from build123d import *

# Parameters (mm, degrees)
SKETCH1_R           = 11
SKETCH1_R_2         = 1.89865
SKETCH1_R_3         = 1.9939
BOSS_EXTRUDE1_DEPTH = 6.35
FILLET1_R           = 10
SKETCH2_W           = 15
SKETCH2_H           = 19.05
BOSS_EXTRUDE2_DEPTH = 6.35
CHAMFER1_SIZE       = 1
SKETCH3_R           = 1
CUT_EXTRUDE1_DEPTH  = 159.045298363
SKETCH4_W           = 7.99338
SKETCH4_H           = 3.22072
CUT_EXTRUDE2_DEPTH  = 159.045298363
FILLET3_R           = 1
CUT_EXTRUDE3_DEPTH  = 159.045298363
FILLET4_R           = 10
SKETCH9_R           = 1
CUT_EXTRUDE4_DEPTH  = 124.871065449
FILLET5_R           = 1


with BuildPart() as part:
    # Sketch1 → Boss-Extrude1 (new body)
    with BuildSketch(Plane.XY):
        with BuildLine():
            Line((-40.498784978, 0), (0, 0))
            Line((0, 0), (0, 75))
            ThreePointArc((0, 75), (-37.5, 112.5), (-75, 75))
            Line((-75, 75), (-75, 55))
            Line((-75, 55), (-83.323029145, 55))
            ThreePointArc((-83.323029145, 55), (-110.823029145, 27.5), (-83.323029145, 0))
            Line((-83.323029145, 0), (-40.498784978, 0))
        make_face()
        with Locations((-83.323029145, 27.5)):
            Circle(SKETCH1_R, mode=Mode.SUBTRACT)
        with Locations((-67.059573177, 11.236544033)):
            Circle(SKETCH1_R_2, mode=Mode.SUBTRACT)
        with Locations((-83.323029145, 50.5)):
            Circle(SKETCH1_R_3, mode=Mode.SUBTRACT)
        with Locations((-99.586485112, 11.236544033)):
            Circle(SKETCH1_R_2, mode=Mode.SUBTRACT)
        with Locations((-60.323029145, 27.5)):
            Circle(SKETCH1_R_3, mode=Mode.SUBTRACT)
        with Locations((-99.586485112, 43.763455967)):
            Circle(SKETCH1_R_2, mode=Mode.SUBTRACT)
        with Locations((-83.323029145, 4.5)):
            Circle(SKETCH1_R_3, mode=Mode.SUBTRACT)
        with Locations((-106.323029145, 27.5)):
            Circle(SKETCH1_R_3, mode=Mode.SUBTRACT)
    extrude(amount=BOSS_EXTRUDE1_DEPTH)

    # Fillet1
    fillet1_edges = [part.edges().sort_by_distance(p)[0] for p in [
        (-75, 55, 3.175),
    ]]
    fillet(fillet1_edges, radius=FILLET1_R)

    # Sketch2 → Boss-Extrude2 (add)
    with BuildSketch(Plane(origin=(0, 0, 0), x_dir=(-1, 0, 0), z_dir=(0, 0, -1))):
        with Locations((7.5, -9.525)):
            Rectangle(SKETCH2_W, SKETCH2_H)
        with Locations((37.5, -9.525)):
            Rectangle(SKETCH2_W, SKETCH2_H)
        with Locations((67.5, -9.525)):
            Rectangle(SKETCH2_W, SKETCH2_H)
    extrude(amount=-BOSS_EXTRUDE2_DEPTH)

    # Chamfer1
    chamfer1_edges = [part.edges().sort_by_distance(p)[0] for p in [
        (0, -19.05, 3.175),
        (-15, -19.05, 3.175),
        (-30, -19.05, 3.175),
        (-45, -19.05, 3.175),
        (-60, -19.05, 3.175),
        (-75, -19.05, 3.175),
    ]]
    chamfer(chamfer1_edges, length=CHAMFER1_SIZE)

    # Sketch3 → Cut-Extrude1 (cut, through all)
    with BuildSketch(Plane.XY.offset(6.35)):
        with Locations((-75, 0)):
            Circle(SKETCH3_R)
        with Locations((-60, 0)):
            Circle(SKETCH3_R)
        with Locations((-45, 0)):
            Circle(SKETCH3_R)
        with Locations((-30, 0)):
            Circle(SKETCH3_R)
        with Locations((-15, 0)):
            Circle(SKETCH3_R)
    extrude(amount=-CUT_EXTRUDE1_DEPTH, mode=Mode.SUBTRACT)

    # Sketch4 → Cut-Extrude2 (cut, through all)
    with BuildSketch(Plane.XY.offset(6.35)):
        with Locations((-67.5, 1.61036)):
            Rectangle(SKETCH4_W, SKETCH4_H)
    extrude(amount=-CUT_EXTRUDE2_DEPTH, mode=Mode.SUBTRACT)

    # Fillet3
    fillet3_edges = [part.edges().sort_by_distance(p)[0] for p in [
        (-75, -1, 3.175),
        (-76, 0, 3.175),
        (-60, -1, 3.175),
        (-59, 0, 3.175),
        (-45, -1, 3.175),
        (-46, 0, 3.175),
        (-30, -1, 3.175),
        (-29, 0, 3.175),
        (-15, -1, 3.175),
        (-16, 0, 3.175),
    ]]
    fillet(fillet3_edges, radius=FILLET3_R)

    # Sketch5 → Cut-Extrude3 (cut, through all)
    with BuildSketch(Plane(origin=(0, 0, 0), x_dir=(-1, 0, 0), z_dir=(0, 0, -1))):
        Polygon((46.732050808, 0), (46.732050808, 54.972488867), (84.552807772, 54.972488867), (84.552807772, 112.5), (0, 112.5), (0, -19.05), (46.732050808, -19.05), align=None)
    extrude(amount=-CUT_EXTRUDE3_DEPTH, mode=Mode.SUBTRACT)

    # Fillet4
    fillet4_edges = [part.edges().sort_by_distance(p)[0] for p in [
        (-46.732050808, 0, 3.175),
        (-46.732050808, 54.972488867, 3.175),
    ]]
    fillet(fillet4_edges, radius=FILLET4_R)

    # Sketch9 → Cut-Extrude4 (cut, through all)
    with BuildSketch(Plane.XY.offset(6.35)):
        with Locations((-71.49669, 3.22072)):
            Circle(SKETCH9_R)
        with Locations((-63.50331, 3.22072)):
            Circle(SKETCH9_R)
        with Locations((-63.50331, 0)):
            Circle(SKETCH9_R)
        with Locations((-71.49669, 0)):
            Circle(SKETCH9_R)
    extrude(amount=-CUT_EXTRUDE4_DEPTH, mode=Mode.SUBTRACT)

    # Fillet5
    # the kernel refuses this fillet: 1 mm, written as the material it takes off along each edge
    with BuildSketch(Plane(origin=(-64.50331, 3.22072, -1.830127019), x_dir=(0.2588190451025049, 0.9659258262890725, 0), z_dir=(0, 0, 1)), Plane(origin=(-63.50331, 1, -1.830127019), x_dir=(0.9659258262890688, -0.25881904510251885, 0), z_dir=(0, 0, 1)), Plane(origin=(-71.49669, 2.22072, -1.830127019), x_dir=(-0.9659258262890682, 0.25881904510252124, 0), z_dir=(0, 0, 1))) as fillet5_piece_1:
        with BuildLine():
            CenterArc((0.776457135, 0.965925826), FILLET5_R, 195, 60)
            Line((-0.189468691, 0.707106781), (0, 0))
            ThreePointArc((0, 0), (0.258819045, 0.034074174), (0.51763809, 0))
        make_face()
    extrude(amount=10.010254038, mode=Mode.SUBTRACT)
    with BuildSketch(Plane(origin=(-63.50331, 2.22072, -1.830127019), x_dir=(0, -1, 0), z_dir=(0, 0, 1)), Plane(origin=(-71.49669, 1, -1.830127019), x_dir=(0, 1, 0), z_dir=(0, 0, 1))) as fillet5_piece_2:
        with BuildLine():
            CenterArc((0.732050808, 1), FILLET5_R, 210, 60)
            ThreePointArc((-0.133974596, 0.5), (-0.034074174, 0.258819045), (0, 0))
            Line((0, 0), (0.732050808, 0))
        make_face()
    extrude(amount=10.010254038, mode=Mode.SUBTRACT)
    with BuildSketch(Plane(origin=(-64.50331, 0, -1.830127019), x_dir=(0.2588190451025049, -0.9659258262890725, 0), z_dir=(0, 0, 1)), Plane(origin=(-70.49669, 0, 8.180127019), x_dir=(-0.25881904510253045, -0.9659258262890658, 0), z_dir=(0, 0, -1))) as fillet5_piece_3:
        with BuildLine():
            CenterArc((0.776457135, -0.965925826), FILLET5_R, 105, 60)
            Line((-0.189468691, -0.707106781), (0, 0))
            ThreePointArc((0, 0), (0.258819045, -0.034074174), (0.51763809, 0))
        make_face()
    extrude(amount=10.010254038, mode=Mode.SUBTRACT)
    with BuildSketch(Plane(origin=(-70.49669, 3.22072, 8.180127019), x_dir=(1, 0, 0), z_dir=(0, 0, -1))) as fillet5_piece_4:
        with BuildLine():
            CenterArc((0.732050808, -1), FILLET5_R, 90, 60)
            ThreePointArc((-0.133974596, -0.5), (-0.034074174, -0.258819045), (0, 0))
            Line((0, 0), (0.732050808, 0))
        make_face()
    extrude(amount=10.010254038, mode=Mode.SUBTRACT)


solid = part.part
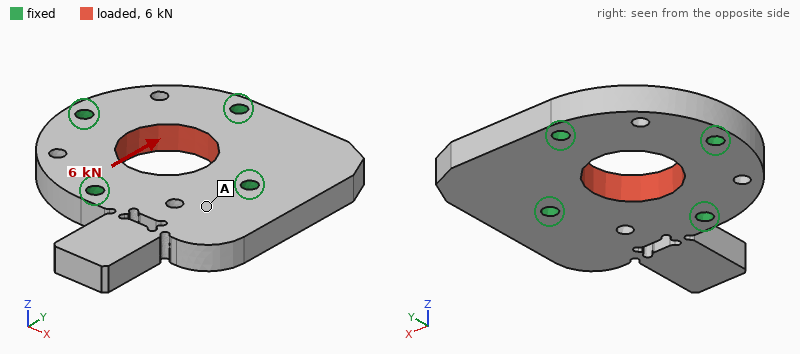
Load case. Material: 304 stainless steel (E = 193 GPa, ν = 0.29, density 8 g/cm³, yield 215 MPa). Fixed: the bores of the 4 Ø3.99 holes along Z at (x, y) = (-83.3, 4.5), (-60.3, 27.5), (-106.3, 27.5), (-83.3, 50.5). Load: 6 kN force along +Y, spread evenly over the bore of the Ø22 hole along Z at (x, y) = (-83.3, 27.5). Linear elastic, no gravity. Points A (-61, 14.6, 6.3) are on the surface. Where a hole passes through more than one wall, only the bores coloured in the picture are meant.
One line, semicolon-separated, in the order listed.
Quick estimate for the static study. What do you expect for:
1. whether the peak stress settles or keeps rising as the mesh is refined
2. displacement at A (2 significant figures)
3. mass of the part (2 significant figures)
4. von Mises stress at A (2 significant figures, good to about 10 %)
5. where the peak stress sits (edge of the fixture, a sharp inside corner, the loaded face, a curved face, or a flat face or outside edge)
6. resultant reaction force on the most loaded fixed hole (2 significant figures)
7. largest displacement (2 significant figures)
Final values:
keeps rising; 0.62 µm; 150 g; 5.6 MPa; edge of the fixture; 1.7 kN; 2.1 µm
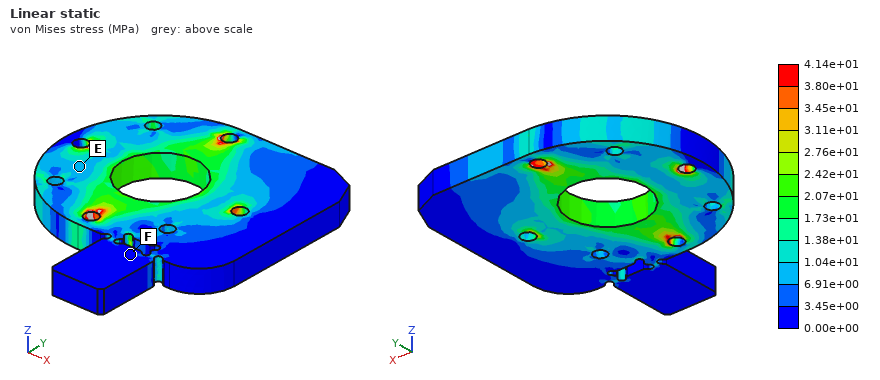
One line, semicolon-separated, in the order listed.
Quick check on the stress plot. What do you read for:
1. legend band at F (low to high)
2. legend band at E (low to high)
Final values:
0.00e+00 to 3.45e+00 MPa; 6.91e+00 to 1.04e+01 MPa
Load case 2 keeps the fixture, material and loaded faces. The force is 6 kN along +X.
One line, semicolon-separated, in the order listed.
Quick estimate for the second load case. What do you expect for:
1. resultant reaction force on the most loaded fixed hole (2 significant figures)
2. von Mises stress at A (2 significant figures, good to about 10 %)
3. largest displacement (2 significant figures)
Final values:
1.8 kN; 6.2 MPa; 2.0 µm
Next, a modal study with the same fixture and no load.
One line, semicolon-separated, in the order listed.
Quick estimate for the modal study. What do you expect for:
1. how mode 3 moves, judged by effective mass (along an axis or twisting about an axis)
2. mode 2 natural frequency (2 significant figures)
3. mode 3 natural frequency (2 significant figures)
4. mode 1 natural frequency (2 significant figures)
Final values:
along Z; 9000 Hz; 10 kHz; 4100 Hz
